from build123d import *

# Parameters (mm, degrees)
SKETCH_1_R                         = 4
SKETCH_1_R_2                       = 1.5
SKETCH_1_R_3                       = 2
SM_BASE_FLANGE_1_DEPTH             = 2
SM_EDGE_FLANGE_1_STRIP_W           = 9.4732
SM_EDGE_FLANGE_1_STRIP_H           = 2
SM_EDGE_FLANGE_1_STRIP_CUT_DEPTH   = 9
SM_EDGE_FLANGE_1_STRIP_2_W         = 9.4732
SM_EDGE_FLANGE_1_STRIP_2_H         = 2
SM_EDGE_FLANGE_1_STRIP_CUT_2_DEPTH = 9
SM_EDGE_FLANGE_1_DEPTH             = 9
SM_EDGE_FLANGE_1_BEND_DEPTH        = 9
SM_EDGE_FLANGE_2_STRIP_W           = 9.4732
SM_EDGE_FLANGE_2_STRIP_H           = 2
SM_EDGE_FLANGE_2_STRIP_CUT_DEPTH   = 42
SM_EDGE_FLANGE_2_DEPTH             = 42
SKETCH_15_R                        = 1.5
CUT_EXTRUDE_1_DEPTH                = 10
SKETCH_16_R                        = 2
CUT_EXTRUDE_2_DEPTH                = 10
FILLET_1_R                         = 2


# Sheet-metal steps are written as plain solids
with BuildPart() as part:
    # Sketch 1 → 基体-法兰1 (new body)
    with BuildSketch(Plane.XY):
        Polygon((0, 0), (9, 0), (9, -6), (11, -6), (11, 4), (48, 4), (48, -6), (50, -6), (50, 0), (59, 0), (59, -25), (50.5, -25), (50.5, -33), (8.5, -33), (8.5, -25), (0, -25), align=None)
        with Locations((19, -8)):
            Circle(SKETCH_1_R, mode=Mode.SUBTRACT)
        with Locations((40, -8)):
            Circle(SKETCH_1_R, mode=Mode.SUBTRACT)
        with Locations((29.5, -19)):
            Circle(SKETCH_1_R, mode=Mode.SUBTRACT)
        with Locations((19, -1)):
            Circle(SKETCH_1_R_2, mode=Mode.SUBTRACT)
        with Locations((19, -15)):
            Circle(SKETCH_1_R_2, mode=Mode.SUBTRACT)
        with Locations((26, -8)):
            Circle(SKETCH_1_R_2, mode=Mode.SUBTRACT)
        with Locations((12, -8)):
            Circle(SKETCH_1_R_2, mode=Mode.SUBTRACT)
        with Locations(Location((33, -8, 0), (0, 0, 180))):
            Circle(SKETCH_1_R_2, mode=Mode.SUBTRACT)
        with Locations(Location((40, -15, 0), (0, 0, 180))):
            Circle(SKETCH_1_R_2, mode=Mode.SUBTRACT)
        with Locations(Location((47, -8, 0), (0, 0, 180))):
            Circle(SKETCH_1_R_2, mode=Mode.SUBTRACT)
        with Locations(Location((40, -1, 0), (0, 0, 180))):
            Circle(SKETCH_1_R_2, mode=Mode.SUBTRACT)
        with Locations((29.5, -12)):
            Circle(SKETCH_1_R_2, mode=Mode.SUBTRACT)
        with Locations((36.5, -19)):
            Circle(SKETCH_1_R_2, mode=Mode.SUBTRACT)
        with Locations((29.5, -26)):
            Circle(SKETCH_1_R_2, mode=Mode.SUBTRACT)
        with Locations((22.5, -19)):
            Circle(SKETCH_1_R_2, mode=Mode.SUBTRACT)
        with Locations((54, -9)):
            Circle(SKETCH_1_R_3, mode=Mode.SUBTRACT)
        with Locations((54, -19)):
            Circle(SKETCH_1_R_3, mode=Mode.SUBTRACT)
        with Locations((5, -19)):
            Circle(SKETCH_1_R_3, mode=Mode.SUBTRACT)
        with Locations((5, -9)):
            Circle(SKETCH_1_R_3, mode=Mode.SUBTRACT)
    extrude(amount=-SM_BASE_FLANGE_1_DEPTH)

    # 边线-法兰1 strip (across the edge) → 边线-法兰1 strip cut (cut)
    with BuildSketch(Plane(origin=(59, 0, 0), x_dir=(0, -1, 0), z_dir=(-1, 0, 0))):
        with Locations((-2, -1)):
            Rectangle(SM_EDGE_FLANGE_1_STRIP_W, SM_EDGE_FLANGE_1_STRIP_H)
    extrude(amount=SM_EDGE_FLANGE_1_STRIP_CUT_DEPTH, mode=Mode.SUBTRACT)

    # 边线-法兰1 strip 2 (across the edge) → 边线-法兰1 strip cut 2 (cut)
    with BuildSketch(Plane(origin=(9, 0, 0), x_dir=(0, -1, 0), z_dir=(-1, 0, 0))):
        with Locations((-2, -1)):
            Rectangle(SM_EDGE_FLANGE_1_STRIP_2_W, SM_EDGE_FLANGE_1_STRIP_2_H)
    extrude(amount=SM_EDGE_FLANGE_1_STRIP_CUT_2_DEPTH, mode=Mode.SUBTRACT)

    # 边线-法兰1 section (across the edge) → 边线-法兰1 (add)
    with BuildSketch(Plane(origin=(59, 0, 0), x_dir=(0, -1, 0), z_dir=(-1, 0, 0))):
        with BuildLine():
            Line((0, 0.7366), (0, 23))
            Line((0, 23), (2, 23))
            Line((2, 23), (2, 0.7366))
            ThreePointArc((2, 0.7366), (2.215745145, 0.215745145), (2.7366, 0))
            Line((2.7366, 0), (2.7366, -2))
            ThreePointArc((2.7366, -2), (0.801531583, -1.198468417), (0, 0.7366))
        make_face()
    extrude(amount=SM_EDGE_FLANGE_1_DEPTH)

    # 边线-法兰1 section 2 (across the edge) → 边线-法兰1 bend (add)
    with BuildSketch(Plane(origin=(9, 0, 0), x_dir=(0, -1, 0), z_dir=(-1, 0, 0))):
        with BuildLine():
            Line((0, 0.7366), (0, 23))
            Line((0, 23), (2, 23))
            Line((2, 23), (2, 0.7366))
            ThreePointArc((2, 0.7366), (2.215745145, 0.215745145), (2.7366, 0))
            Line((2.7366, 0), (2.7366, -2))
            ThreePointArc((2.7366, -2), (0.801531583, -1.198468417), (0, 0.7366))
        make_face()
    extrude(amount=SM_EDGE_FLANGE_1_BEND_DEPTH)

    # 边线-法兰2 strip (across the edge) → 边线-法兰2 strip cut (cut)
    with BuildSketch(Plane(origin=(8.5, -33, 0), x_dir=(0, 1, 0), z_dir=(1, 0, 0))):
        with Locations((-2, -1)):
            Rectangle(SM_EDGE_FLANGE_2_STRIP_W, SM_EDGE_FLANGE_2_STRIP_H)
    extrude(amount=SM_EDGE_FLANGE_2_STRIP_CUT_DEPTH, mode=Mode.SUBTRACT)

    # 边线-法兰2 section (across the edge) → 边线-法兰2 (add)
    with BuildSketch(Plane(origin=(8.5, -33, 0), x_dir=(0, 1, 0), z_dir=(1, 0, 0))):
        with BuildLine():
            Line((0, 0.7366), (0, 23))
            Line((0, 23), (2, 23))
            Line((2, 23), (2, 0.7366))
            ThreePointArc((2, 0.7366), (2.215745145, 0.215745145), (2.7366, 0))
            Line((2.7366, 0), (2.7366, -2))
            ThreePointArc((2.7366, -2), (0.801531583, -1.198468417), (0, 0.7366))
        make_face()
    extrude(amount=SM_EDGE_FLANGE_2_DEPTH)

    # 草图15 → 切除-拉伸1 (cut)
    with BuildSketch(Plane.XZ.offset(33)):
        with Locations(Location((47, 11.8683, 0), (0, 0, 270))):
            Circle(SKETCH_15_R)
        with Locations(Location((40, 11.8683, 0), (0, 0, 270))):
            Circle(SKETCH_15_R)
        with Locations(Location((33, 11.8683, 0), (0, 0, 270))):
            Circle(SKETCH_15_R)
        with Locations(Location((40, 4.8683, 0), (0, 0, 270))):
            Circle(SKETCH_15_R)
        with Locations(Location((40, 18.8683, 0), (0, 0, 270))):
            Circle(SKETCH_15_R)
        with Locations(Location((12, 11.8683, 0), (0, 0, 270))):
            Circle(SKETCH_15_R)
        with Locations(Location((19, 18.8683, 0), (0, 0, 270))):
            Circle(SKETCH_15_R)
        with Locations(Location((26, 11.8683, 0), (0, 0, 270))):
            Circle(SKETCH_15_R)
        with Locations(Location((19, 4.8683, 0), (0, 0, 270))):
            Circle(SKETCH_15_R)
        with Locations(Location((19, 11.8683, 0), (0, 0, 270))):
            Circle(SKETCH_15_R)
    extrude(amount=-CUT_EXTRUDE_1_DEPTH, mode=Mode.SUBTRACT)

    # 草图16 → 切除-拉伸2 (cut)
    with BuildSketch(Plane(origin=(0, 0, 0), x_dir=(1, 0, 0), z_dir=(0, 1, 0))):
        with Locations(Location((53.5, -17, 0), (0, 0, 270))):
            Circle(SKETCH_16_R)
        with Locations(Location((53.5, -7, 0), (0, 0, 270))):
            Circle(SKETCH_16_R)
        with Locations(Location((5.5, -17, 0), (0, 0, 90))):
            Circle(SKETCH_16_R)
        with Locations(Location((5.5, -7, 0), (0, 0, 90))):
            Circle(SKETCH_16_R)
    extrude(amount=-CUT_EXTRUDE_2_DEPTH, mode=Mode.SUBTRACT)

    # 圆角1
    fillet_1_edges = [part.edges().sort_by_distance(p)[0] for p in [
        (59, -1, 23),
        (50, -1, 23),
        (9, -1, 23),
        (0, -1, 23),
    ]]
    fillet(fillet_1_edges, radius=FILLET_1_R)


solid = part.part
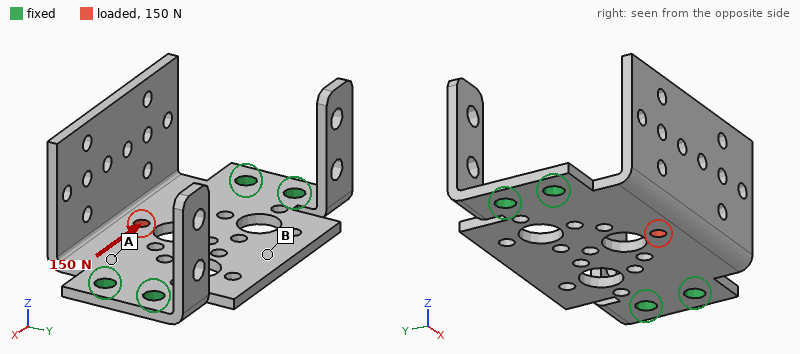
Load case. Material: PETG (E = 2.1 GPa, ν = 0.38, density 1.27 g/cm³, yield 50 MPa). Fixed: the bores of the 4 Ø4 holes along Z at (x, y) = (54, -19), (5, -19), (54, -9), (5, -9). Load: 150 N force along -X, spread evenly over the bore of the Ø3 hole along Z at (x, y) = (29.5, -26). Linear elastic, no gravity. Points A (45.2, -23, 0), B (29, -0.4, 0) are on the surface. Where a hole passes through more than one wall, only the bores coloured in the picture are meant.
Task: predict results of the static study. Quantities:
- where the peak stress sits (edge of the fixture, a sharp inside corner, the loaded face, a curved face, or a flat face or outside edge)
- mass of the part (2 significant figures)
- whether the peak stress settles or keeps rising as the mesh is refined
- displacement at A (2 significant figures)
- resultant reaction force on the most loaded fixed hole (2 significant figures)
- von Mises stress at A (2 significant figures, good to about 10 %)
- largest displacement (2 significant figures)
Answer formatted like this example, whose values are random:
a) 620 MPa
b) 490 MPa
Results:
a) a sharp inside corner
b) 7.3 g
c) keeps rising
d) 17 µm
e) 65 N
f) 3.6 MPa
g) 53 µm
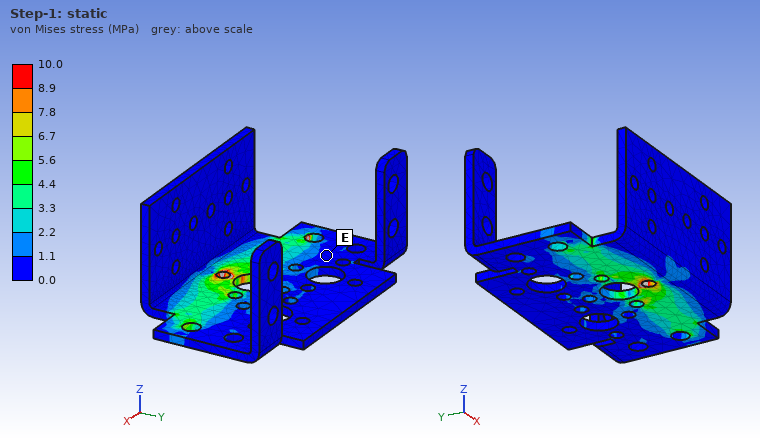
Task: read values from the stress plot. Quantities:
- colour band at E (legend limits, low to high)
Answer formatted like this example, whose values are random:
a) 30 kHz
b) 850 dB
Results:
a) 0.0 to 1.1 MPa
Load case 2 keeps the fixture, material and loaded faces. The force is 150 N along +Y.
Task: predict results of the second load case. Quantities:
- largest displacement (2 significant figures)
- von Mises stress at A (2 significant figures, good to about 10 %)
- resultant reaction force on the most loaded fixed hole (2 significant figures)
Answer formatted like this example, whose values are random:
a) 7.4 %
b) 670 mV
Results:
a) 0.12 mm
b) 3.0 MPa
c) 53 N
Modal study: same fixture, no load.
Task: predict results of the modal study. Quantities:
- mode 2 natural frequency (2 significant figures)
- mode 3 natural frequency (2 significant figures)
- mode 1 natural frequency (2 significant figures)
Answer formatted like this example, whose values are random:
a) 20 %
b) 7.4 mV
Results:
a) 540 Hz
b) 540 Hz
c) 360 Hz
